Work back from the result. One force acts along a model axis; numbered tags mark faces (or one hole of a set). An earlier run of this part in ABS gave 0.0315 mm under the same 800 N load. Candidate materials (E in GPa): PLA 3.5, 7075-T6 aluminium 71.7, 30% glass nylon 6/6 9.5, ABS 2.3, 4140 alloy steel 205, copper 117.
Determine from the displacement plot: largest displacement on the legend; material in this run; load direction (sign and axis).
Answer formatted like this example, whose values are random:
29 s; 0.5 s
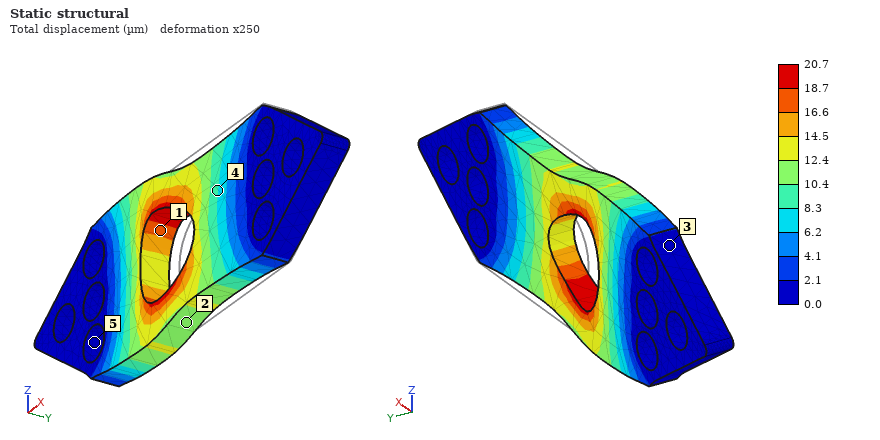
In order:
20.7 µm; PLA; -X
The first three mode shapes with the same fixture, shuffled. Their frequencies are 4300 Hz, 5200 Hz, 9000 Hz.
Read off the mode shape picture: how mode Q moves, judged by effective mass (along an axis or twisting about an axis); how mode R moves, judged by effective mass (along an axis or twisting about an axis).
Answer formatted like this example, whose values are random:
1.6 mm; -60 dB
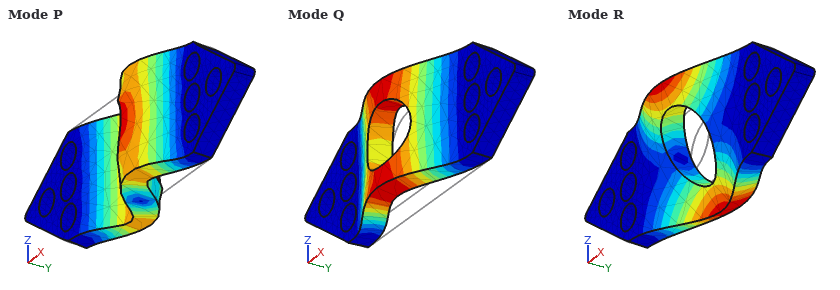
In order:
along Y; twisting about X
